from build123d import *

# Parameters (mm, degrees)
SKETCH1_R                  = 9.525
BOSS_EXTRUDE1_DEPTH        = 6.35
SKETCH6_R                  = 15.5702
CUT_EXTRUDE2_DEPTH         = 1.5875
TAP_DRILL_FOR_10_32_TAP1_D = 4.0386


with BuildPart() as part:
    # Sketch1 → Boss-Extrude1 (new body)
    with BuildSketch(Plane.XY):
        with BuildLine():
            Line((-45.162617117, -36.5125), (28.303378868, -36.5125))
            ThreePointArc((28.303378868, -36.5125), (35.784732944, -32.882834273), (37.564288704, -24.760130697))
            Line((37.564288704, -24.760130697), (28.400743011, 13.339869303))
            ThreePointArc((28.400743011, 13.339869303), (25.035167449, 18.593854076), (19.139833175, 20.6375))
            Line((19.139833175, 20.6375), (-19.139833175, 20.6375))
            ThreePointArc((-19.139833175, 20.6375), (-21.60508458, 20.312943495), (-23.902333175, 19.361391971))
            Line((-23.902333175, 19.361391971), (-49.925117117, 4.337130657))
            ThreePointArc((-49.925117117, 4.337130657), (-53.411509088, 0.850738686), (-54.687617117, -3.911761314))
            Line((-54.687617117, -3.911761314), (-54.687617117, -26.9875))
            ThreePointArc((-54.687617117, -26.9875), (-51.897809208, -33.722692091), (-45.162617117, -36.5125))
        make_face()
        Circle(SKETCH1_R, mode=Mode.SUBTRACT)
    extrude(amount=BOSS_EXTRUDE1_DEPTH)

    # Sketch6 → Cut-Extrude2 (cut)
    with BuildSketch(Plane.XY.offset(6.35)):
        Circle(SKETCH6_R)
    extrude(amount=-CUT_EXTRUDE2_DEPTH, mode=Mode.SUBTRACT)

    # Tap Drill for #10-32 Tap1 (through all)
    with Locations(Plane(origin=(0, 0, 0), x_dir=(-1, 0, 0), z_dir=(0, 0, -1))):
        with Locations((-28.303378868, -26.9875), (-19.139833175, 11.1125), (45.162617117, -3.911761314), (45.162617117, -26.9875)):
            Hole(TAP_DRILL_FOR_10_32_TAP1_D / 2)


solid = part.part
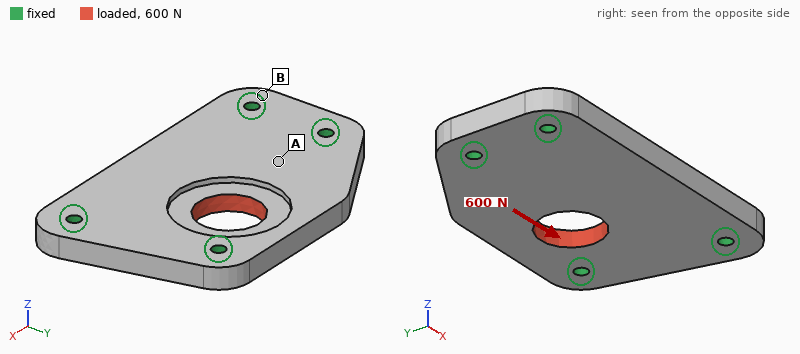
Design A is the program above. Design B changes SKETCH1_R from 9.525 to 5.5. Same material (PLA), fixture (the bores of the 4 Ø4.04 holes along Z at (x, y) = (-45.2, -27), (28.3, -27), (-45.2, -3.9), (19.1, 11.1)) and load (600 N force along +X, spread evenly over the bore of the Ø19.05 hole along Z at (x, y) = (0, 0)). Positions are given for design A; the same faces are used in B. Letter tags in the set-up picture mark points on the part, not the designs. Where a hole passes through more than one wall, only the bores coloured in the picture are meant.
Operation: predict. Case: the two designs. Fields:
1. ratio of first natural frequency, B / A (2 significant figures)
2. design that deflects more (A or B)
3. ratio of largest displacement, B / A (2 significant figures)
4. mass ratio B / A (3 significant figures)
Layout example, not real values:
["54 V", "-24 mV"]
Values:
["1.00", "B", "1.2", "1.03"]
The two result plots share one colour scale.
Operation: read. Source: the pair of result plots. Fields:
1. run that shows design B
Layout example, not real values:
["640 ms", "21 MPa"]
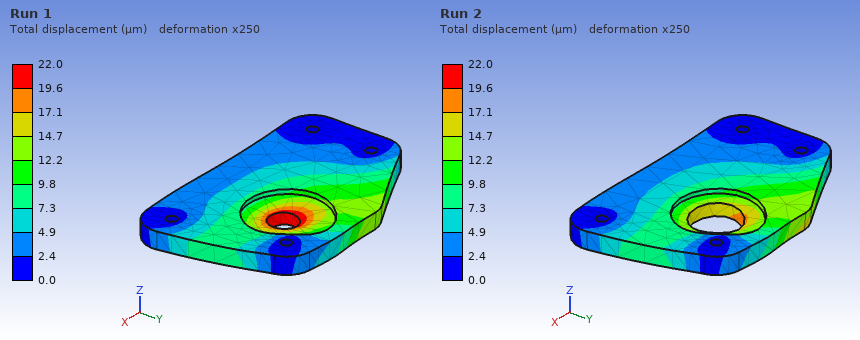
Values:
["Run 1"]
